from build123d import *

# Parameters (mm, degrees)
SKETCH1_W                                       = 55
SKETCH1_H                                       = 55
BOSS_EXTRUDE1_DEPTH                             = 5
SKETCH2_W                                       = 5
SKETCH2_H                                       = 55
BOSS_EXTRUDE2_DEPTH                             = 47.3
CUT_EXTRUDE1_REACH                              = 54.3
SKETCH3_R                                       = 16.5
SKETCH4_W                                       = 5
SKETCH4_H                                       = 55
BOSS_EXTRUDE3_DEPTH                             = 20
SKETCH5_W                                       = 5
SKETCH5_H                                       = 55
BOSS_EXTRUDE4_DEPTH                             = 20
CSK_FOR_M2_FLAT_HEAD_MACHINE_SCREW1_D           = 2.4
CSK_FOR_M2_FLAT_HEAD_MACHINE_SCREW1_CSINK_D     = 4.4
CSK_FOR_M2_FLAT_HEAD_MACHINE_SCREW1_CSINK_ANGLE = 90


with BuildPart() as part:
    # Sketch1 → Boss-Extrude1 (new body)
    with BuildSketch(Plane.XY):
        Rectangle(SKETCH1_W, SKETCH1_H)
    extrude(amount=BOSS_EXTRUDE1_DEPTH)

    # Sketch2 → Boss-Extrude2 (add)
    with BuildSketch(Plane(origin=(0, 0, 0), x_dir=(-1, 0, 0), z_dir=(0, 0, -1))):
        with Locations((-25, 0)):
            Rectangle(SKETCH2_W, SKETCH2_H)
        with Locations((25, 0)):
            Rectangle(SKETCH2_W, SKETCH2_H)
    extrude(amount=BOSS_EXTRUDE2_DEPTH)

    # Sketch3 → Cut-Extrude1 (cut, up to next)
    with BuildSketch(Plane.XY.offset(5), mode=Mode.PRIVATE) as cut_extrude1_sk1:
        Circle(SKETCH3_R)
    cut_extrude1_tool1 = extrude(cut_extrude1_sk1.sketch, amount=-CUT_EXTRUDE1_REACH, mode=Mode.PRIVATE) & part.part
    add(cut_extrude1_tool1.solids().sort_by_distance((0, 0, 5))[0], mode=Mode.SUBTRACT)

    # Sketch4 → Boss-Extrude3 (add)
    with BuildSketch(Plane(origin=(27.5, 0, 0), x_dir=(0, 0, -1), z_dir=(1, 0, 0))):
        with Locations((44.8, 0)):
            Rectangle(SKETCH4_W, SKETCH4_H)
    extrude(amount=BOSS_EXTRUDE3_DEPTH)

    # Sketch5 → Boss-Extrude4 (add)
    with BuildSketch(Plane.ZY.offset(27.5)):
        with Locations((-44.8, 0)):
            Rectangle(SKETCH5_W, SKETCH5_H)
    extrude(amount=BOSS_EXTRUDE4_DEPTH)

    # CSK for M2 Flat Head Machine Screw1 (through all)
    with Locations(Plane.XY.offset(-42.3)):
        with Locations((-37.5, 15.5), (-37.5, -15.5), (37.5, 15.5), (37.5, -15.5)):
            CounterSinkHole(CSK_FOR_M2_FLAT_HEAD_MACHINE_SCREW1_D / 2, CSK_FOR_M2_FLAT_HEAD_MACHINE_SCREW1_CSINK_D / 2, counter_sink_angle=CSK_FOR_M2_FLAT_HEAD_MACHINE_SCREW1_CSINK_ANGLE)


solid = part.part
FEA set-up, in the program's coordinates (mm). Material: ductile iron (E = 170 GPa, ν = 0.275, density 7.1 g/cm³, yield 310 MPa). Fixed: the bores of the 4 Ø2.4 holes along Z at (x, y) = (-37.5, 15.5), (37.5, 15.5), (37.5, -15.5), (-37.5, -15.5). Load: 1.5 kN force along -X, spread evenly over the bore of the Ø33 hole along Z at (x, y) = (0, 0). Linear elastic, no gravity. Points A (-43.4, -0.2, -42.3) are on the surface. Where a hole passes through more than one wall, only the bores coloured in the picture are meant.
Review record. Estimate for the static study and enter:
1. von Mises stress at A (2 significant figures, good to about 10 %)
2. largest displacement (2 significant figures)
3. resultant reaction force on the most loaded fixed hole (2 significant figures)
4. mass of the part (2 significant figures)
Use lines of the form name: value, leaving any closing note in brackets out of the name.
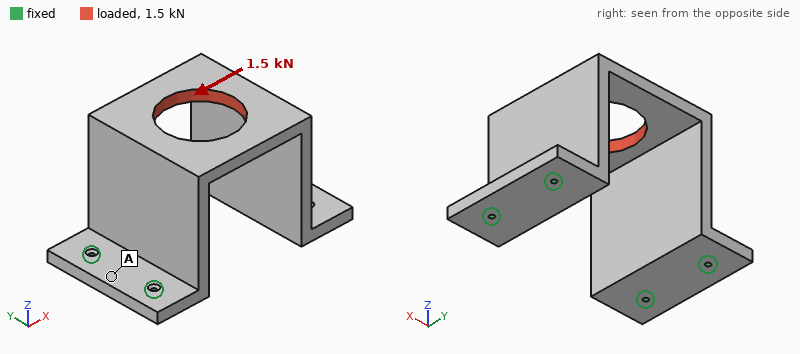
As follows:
von Mises stress at A: 10.0 MPa
largest displacement: 0.15 mm
resultant reaction force on the most loaded fixed hole: 530 N
mass of the part: 340 g
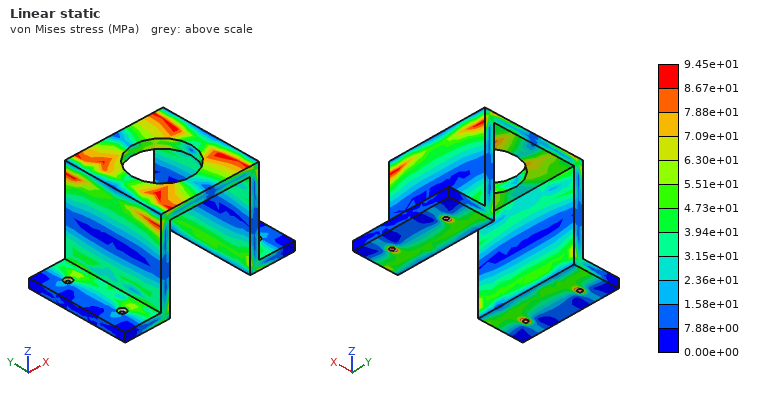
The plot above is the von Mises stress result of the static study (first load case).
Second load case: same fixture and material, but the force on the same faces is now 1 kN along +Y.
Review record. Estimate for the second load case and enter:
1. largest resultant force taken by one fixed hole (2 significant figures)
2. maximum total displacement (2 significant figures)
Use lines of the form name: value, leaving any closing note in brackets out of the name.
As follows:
largest resultant force taken by one fixed hole: 780 N
maximum total displacement: 37 µm
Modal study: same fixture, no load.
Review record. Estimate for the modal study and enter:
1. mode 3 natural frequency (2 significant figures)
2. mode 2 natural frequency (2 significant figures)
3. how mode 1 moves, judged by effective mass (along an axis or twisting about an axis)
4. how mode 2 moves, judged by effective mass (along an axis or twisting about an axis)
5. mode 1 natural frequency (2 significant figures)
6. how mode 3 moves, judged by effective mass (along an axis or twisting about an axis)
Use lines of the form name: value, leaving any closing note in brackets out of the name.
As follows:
mode 3 natural frequency: 2400 Hz
mode 2 natural frequency: 2300 Hz
how mode 1 moves, judged by effective mass: along X
how mode 2 moves, judged by effective mass: along Y
mode 1 natural frequency: 1400 Hz
how mode 3 moves, judged by effective mass: twisting about Z
